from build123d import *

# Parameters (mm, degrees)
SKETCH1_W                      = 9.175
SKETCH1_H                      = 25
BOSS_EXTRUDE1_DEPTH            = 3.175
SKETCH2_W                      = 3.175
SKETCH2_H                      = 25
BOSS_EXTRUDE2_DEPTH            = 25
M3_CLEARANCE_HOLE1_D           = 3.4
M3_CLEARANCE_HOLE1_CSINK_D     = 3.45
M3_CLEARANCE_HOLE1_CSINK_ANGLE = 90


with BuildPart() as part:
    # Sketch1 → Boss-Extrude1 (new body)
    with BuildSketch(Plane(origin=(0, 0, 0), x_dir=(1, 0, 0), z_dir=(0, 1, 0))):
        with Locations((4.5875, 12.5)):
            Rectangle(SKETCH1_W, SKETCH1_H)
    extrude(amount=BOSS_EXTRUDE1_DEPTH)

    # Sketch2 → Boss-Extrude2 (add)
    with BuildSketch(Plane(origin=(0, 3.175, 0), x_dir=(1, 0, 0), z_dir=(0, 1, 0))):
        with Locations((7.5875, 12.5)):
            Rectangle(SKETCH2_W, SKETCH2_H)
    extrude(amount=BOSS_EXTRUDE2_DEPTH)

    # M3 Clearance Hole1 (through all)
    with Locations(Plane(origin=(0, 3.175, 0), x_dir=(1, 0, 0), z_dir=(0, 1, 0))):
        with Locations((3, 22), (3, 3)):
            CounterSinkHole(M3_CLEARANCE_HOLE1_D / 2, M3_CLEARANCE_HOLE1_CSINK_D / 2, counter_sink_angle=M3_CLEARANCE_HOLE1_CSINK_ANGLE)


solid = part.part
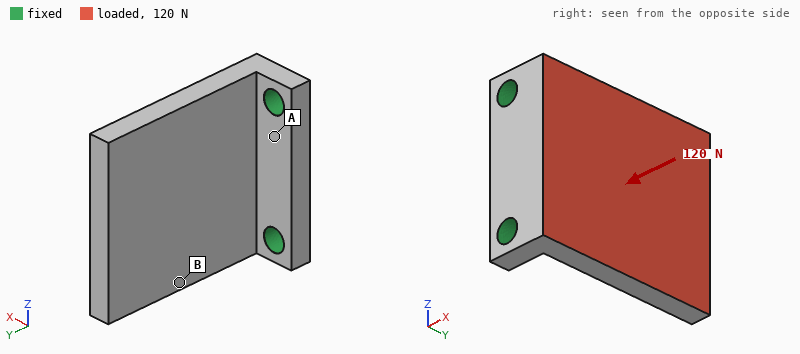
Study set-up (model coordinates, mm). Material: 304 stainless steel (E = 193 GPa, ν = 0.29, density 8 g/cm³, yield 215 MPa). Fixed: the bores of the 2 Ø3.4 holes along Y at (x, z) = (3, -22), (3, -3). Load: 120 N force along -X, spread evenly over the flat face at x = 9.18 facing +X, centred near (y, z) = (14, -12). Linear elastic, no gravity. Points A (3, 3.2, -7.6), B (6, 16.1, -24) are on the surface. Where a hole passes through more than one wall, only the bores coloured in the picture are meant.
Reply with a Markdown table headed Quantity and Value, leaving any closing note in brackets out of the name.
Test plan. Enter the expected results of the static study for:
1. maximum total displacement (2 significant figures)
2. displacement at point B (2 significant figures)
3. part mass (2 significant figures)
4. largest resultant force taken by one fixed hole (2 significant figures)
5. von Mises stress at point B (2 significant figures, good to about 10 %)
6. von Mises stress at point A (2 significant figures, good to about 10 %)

| Quantity | Value |
|---|---|
| maximum total displacement | 32 µm |
| displacement at point B | 14 µm |
| part mass | 21 g |
| largest resultant force taken by one fixed hole | 63 N |
| von Mises stress at point B | 7.2 MPa |
| von Mises stress at point A | 18 MPa |
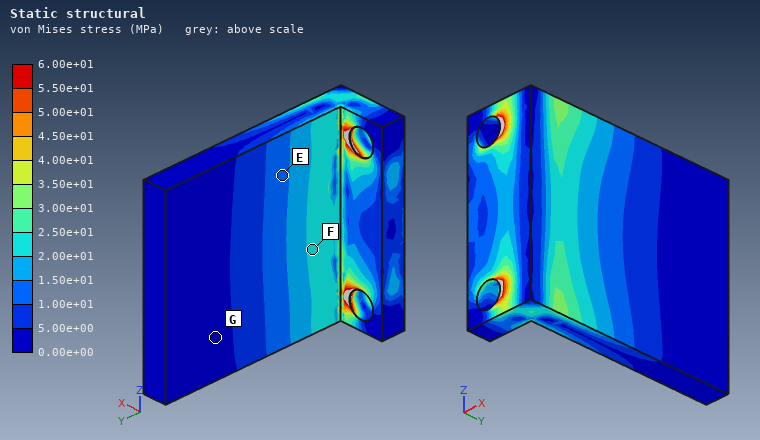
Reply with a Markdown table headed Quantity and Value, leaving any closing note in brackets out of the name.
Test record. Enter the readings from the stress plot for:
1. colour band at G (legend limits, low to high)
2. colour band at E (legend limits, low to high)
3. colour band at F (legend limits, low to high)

| Quantity | Value |
|---|---|
| colour band at G | 0.00e+00 to 5.00e+00 MPa |
| colour band at E | 1.00e+01 to 1.50e+01 MPa |
| colour band at F | 2.00e+01 to 2.50e+01 MPa |
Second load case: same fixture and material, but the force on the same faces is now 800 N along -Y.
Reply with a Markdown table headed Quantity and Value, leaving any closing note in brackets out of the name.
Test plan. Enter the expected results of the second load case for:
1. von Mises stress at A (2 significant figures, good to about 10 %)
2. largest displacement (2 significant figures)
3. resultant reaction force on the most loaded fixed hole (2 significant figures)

| Quantity | Value |
|---|---|
| von Mises stress at A | 37 MPa |
| largest displacement | 50 µm |
| resultant reaction force on the most loaded fixed hole | 400 N |
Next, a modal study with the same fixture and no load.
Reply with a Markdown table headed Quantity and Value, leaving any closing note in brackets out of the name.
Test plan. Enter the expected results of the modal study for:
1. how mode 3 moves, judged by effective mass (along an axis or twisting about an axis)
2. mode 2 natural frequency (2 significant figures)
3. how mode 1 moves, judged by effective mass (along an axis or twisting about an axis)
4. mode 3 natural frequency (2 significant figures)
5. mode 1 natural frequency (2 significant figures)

| Quantity | Value |
|---|---|
| how mode 3 moves, judged by effective mass | along Z |
| mode 2 natural frequency | 8100 Hz |
| how mode 1 moves, judged by effective mass | along X |
| mode 3 natural frequency | 12 kHz |
| mode 1 natural frequency | 2900 Hz |
